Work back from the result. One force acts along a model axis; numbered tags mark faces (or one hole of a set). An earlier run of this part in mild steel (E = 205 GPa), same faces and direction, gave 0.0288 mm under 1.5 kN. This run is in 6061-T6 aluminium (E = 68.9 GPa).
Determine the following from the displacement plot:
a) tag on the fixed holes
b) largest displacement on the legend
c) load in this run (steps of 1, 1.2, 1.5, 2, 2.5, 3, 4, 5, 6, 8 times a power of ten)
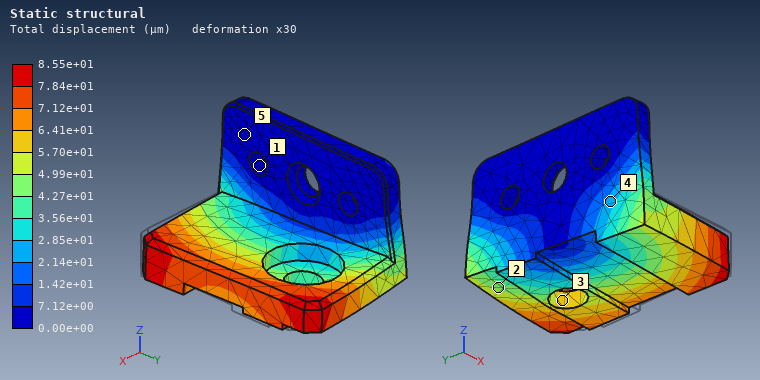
1
8.55e+01 µm
1.5 kN
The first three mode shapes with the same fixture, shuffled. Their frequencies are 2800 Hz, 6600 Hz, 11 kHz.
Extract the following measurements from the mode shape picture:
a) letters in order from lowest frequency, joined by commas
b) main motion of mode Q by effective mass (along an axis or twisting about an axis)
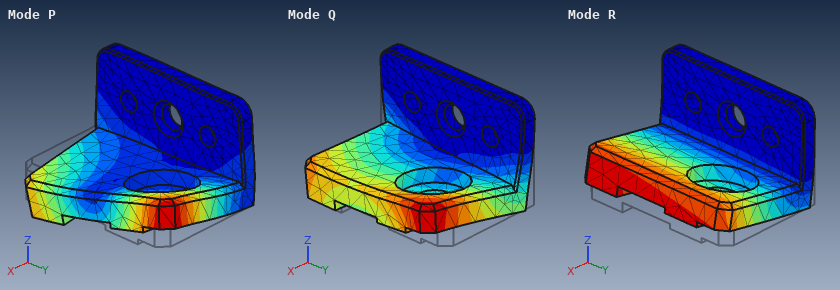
R, Q, P
along Y
